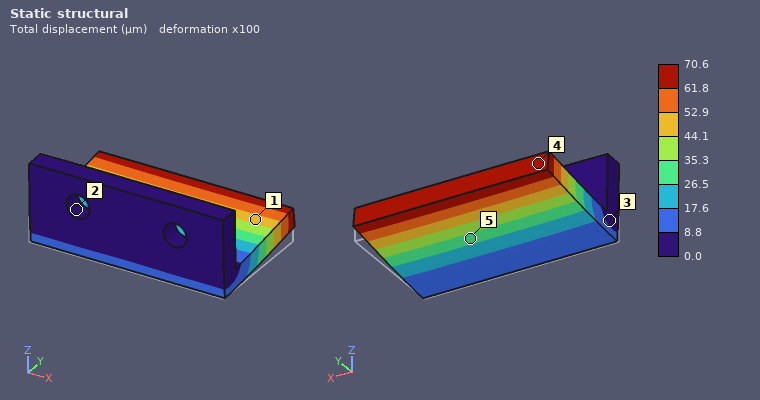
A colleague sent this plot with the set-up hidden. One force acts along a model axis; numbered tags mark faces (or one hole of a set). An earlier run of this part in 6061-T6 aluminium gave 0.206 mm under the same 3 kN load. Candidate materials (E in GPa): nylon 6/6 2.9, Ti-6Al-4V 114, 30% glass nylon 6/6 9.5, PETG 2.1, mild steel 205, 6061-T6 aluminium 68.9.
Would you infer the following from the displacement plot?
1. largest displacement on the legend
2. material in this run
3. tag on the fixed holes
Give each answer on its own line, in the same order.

70.6 µm
mild steel
2
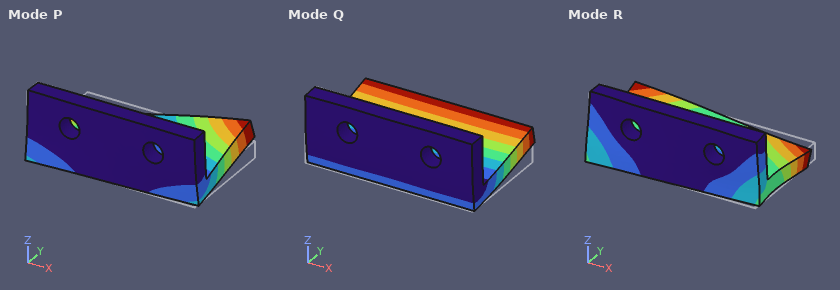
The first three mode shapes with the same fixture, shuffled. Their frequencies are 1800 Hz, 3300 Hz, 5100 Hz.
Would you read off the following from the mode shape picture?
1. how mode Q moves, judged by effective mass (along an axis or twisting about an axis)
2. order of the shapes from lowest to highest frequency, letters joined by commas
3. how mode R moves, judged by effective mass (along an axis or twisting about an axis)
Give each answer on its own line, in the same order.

along Z
Q, P, R
along X
